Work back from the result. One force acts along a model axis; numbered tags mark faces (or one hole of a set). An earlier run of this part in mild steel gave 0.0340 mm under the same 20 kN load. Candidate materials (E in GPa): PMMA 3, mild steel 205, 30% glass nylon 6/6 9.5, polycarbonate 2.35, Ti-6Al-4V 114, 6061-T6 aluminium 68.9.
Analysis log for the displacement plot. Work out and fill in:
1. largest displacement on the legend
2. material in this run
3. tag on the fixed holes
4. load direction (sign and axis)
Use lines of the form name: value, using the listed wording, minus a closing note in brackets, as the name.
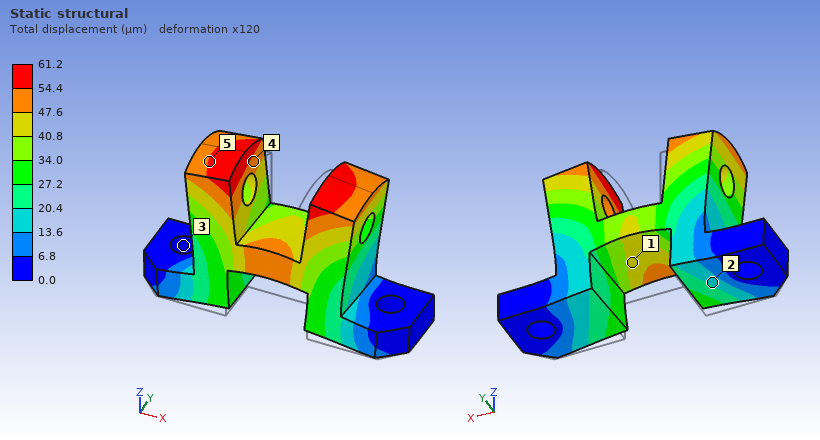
largest displacement on the legend: 61.2 µm
material in this run: Ti-6Al-4V
tag on the fixed holes: 3
load direction: +Z
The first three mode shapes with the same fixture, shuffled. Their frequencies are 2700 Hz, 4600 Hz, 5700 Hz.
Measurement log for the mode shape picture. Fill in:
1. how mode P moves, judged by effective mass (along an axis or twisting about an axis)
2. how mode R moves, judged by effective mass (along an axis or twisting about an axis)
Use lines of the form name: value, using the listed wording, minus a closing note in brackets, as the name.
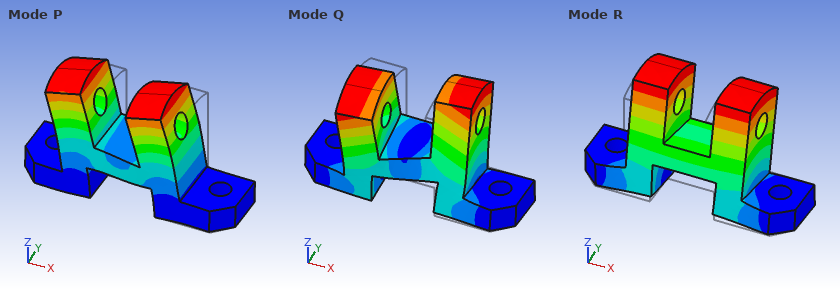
how mode P moves, judged by effective mass: along X
how mode R moves, judged by effective mass: along Y
